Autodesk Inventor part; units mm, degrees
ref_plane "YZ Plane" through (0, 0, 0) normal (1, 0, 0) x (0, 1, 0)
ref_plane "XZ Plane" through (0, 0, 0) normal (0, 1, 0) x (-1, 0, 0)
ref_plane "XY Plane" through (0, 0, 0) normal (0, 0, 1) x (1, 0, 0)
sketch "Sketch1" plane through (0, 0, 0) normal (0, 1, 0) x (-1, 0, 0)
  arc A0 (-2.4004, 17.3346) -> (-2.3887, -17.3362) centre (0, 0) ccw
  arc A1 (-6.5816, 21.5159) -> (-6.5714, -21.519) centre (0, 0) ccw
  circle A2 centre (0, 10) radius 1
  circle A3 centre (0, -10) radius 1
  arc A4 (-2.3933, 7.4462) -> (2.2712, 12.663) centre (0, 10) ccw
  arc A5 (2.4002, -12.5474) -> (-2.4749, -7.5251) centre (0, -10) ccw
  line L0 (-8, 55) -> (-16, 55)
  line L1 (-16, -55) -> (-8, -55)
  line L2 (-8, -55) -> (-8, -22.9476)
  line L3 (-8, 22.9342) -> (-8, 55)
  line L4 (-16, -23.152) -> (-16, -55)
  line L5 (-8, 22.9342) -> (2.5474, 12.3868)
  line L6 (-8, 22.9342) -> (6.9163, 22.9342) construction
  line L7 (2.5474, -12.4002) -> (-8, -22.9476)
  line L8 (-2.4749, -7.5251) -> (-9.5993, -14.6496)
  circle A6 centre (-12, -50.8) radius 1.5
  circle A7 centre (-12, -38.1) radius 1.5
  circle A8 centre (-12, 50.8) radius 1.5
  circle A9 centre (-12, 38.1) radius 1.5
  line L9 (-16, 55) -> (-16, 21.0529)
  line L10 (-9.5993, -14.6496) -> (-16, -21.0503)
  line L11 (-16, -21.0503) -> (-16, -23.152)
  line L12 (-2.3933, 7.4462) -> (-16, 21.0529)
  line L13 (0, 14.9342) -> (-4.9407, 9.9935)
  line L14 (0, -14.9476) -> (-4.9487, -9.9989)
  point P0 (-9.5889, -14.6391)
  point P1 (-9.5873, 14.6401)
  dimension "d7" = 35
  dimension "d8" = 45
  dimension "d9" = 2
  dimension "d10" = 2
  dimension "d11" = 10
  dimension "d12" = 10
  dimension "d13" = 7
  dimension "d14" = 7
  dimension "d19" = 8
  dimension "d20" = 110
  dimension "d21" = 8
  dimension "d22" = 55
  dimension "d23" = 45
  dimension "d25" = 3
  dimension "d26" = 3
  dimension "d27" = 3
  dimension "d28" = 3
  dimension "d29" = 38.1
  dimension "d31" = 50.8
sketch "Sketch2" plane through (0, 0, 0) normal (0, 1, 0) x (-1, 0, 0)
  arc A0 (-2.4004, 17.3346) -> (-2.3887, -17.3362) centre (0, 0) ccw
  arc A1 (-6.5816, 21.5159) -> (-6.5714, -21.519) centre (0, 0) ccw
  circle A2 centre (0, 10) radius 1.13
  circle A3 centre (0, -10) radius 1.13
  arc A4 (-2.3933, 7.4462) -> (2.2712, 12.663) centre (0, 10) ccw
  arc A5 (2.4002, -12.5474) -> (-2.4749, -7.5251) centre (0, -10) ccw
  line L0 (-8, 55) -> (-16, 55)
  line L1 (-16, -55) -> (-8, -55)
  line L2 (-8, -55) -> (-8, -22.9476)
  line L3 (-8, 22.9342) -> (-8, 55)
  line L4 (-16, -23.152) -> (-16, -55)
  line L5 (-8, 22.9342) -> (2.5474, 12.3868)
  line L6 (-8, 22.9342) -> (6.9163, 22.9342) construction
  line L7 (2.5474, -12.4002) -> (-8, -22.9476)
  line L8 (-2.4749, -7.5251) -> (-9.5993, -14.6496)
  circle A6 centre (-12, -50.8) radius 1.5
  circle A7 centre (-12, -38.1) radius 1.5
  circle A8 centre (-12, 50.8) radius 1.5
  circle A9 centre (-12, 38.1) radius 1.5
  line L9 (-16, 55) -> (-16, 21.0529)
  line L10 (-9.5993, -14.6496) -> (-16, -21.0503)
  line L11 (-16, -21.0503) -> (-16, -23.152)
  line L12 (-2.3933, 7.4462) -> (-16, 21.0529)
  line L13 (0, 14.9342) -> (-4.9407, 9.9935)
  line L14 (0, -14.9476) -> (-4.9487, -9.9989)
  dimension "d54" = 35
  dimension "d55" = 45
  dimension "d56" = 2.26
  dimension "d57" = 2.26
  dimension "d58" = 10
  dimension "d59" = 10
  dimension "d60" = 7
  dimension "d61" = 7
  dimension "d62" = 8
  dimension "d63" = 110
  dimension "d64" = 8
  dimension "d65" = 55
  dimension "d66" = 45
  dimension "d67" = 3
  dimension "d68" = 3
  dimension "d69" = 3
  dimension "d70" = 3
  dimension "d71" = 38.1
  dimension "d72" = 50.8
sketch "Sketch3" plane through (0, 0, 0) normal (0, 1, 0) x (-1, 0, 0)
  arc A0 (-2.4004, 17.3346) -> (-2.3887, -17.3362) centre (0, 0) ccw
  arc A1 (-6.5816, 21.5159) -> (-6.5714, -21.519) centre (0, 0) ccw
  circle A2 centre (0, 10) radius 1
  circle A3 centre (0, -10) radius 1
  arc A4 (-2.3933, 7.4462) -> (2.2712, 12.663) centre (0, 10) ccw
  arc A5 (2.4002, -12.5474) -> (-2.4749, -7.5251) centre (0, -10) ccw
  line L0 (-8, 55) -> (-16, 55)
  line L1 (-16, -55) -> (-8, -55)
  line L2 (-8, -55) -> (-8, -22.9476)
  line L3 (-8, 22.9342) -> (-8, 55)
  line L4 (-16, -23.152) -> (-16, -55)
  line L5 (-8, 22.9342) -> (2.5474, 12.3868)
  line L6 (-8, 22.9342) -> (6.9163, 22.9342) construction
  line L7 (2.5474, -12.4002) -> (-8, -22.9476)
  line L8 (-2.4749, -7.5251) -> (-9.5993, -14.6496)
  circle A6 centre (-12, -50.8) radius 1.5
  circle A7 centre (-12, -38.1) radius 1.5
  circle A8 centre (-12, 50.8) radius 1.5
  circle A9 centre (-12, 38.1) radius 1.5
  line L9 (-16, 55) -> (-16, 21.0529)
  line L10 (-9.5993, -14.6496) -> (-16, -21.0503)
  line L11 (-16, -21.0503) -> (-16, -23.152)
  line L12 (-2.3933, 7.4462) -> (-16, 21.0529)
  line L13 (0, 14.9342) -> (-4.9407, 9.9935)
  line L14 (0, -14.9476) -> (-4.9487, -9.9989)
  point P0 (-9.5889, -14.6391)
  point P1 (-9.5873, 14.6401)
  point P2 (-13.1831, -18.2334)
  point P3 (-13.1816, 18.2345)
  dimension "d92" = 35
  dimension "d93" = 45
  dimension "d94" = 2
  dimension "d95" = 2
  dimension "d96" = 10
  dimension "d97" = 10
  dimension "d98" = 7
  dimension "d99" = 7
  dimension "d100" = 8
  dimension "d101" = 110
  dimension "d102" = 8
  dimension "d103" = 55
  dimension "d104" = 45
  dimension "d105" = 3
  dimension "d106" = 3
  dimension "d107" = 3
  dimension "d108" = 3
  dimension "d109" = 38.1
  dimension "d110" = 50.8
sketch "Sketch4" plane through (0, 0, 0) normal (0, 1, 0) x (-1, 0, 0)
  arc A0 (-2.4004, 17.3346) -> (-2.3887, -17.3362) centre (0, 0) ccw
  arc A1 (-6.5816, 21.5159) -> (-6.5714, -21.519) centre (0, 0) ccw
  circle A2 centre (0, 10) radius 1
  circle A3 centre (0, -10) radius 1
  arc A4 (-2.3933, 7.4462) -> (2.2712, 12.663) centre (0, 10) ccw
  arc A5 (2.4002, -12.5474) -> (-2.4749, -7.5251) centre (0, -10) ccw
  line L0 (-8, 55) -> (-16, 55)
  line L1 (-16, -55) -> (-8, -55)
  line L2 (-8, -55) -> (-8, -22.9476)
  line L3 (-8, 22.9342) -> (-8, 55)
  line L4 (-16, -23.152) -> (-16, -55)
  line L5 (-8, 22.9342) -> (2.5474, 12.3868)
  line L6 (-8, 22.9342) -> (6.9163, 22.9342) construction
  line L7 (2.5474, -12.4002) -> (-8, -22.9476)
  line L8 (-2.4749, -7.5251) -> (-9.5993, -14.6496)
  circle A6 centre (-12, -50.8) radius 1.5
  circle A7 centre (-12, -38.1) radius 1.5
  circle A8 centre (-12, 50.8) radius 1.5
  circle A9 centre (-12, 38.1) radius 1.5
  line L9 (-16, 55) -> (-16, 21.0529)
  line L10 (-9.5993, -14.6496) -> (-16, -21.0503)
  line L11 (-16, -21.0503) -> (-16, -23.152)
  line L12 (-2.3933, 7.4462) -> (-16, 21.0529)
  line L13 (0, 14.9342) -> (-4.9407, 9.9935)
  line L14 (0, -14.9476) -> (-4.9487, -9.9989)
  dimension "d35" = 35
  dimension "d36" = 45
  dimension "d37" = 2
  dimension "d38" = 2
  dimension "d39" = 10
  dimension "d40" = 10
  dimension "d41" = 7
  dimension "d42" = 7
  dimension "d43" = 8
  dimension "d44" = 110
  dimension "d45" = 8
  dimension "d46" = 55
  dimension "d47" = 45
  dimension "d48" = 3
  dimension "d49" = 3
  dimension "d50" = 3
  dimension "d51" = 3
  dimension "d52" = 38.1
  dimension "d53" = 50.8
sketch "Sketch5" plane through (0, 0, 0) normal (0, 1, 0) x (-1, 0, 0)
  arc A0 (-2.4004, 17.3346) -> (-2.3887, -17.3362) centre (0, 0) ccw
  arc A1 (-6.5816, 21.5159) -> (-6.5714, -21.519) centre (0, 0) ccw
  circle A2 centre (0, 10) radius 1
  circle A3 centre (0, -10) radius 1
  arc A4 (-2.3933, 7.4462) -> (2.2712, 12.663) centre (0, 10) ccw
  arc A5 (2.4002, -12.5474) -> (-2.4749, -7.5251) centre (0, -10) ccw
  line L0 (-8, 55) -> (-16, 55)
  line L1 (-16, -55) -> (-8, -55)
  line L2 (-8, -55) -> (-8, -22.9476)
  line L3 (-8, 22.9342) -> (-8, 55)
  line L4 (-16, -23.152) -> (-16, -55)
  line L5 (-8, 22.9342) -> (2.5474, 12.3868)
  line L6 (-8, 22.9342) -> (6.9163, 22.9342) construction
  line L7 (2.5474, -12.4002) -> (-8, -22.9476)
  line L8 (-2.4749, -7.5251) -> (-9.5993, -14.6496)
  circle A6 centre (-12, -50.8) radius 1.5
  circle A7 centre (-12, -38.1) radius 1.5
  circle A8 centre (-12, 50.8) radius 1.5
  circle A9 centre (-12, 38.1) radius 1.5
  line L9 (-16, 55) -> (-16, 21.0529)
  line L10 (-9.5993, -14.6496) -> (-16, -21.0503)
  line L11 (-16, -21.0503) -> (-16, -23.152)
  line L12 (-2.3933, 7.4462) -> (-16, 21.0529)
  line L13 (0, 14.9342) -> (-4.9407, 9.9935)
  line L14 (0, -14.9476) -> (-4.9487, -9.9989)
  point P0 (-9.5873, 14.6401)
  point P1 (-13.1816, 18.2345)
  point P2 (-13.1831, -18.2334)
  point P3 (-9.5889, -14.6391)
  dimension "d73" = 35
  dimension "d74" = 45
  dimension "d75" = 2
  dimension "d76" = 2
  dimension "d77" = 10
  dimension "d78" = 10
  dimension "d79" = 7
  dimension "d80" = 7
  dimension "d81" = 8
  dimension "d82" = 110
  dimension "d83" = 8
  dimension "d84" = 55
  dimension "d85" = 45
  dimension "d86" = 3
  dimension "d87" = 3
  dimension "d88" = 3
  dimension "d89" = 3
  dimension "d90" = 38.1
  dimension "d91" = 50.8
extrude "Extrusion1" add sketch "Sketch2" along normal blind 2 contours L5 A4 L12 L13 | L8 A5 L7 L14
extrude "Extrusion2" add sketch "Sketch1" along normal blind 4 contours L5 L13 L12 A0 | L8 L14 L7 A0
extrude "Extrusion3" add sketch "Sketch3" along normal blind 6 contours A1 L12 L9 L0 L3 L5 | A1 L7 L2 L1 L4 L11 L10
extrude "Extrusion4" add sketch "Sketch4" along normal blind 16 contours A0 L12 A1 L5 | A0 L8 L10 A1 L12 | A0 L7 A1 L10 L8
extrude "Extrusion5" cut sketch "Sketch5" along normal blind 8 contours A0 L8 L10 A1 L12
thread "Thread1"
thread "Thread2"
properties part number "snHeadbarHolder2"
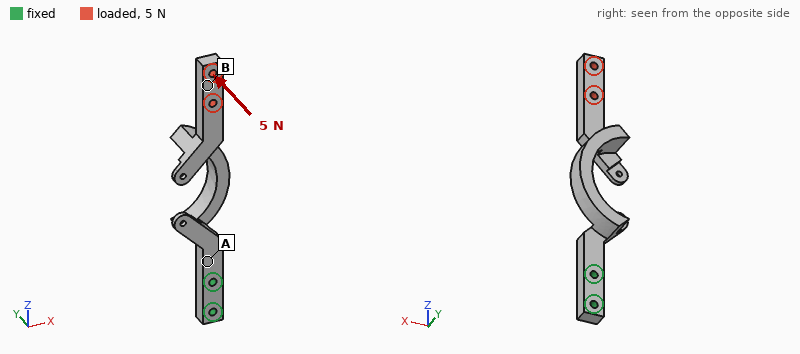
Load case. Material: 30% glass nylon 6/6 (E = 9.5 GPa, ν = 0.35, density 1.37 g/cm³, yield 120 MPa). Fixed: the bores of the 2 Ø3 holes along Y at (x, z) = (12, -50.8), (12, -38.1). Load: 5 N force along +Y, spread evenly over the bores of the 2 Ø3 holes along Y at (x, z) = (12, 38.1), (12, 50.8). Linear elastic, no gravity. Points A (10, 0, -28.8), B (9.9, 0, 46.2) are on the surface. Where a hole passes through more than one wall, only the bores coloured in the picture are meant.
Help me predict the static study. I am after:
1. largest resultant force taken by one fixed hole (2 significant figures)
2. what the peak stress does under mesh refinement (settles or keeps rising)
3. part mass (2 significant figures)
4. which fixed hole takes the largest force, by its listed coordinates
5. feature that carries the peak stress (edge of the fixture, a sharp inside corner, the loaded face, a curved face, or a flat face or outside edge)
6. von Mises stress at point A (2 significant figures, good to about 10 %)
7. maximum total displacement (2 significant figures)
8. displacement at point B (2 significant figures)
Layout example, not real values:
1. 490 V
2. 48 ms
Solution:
1. 8.7 N
2. keeps rising
3. 8.8 g
4. (12, -38.1)
5. a sharp inside corner
6. 7.8 MPa
7. 1.2 mm
8. 1.0 mm
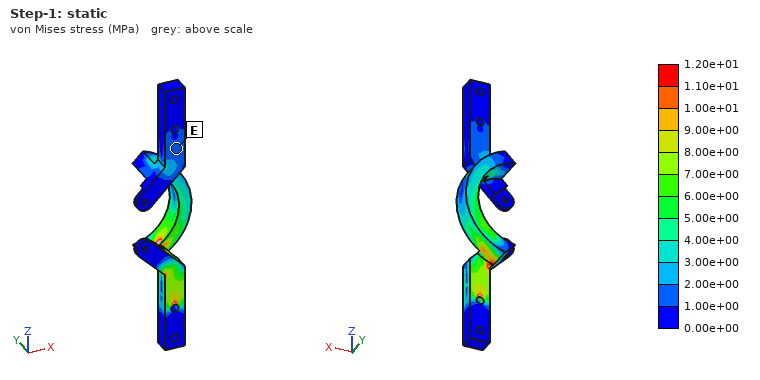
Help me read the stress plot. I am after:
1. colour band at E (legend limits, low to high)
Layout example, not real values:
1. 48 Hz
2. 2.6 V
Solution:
1. 1.00e+00 to 2.00e+00 MPa
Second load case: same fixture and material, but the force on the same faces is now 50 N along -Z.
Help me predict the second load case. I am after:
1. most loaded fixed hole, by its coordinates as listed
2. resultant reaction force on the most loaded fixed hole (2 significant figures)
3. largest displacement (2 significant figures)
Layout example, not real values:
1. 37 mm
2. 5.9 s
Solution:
1. (12, -38.1)
2. 47 N
3. 1.2 mm
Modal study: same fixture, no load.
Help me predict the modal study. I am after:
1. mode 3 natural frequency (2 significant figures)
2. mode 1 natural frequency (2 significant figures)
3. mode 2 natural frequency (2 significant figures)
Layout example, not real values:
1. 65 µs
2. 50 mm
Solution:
1. 1000 Hz
2. 240 Hz
3. 240 Hz
